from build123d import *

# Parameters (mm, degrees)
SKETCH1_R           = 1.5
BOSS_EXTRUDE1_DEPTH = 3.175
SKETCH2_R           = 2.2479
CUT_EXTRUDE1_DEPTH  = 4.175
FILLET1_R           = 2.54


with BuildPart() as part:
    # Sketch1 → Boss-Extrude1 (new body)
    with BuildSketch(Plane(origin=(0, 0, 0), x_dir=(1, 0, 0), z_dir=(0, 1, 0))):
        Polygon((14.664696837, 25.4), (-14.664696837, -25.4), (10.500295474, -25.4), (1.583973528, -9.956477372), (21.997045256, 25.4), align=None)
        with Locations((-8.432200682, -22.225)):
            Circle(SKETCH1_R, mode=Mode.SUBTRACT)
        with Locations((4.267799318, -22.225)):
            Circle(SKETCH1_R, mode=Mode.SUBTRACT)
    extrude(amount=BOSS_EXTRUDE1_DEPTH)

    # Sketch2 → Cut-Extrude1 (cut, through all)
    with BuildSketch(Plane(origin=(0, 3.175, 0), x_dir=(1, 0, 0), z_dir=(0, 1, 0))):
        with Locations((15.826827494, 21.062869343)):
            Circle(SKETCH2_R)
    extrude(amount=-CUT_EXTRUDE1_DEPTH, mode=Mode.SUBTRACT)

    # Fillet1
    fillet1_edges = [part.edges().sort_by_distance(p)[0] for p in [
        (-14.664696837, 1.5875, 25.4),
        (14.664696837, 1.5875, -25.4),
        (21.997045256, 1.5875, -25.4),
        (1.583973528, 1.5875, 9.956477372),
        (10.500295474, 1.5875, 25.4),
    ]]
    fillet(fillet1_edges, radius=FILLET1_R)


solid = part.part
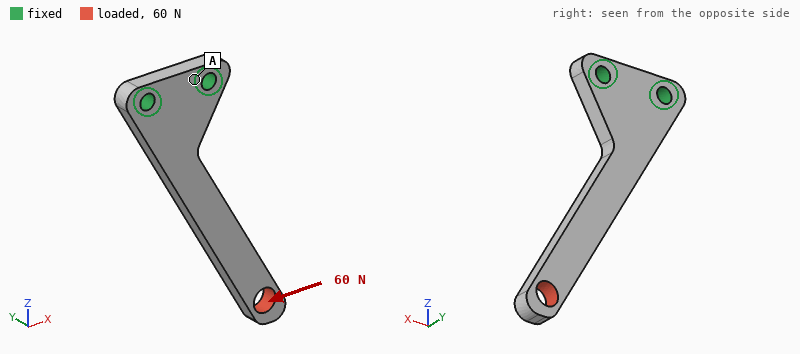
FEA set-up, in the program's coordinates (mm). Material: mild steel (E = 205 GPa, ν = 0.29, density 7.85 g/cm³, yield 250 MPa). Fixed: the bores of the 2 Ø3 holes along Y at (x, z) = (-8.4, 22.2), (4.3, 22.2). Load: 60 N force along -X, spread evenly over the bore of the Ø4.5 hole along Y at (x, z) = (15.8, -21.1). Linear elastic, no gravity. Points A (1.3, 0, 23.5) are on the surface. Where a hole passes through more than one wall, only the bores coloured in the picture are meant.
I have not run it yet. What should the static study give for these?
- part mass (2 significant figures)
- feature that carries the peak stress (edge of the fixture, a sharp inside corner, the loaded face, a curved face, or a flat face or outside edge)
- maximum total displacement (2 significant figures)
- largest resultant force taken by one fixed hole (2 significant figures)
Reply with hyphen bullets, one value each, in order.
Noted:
- 12 g
- a curved face
- 83 µm
- 200 N
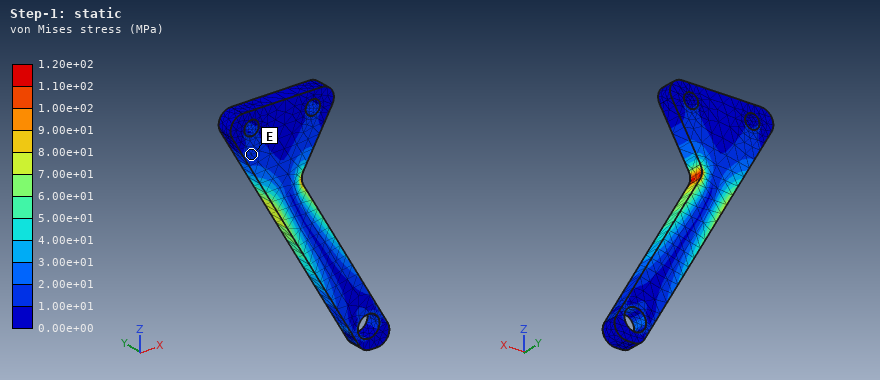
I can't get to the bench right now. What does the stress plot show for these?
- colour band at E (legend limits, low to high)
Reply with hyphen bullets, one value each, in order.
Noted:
- 1.00e+01 to 2.00e+01 MPa
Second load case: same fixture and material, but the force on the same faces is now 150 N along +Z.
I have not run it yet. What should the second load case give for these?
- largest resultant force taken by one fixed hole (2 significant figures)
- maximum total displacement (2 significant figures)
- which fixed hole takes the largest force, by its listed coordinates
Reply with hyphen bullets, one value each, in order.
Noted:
- 280 N
- 0.12 mm
- (4.3, 22.2)
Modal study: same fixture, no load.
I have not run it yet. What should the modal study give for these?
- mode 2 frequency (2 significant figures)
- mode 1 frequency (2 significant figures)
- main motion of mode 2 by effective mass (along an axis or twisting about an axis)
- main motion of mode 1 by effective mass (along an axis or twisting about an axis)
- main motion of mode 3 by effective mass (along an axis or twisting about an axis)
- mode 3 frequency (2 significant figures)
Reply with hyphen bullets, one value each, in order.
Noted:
- 3200 Hz
- 1300 Hz
- along X
- along Y
- along Y
- 7000 Hz
